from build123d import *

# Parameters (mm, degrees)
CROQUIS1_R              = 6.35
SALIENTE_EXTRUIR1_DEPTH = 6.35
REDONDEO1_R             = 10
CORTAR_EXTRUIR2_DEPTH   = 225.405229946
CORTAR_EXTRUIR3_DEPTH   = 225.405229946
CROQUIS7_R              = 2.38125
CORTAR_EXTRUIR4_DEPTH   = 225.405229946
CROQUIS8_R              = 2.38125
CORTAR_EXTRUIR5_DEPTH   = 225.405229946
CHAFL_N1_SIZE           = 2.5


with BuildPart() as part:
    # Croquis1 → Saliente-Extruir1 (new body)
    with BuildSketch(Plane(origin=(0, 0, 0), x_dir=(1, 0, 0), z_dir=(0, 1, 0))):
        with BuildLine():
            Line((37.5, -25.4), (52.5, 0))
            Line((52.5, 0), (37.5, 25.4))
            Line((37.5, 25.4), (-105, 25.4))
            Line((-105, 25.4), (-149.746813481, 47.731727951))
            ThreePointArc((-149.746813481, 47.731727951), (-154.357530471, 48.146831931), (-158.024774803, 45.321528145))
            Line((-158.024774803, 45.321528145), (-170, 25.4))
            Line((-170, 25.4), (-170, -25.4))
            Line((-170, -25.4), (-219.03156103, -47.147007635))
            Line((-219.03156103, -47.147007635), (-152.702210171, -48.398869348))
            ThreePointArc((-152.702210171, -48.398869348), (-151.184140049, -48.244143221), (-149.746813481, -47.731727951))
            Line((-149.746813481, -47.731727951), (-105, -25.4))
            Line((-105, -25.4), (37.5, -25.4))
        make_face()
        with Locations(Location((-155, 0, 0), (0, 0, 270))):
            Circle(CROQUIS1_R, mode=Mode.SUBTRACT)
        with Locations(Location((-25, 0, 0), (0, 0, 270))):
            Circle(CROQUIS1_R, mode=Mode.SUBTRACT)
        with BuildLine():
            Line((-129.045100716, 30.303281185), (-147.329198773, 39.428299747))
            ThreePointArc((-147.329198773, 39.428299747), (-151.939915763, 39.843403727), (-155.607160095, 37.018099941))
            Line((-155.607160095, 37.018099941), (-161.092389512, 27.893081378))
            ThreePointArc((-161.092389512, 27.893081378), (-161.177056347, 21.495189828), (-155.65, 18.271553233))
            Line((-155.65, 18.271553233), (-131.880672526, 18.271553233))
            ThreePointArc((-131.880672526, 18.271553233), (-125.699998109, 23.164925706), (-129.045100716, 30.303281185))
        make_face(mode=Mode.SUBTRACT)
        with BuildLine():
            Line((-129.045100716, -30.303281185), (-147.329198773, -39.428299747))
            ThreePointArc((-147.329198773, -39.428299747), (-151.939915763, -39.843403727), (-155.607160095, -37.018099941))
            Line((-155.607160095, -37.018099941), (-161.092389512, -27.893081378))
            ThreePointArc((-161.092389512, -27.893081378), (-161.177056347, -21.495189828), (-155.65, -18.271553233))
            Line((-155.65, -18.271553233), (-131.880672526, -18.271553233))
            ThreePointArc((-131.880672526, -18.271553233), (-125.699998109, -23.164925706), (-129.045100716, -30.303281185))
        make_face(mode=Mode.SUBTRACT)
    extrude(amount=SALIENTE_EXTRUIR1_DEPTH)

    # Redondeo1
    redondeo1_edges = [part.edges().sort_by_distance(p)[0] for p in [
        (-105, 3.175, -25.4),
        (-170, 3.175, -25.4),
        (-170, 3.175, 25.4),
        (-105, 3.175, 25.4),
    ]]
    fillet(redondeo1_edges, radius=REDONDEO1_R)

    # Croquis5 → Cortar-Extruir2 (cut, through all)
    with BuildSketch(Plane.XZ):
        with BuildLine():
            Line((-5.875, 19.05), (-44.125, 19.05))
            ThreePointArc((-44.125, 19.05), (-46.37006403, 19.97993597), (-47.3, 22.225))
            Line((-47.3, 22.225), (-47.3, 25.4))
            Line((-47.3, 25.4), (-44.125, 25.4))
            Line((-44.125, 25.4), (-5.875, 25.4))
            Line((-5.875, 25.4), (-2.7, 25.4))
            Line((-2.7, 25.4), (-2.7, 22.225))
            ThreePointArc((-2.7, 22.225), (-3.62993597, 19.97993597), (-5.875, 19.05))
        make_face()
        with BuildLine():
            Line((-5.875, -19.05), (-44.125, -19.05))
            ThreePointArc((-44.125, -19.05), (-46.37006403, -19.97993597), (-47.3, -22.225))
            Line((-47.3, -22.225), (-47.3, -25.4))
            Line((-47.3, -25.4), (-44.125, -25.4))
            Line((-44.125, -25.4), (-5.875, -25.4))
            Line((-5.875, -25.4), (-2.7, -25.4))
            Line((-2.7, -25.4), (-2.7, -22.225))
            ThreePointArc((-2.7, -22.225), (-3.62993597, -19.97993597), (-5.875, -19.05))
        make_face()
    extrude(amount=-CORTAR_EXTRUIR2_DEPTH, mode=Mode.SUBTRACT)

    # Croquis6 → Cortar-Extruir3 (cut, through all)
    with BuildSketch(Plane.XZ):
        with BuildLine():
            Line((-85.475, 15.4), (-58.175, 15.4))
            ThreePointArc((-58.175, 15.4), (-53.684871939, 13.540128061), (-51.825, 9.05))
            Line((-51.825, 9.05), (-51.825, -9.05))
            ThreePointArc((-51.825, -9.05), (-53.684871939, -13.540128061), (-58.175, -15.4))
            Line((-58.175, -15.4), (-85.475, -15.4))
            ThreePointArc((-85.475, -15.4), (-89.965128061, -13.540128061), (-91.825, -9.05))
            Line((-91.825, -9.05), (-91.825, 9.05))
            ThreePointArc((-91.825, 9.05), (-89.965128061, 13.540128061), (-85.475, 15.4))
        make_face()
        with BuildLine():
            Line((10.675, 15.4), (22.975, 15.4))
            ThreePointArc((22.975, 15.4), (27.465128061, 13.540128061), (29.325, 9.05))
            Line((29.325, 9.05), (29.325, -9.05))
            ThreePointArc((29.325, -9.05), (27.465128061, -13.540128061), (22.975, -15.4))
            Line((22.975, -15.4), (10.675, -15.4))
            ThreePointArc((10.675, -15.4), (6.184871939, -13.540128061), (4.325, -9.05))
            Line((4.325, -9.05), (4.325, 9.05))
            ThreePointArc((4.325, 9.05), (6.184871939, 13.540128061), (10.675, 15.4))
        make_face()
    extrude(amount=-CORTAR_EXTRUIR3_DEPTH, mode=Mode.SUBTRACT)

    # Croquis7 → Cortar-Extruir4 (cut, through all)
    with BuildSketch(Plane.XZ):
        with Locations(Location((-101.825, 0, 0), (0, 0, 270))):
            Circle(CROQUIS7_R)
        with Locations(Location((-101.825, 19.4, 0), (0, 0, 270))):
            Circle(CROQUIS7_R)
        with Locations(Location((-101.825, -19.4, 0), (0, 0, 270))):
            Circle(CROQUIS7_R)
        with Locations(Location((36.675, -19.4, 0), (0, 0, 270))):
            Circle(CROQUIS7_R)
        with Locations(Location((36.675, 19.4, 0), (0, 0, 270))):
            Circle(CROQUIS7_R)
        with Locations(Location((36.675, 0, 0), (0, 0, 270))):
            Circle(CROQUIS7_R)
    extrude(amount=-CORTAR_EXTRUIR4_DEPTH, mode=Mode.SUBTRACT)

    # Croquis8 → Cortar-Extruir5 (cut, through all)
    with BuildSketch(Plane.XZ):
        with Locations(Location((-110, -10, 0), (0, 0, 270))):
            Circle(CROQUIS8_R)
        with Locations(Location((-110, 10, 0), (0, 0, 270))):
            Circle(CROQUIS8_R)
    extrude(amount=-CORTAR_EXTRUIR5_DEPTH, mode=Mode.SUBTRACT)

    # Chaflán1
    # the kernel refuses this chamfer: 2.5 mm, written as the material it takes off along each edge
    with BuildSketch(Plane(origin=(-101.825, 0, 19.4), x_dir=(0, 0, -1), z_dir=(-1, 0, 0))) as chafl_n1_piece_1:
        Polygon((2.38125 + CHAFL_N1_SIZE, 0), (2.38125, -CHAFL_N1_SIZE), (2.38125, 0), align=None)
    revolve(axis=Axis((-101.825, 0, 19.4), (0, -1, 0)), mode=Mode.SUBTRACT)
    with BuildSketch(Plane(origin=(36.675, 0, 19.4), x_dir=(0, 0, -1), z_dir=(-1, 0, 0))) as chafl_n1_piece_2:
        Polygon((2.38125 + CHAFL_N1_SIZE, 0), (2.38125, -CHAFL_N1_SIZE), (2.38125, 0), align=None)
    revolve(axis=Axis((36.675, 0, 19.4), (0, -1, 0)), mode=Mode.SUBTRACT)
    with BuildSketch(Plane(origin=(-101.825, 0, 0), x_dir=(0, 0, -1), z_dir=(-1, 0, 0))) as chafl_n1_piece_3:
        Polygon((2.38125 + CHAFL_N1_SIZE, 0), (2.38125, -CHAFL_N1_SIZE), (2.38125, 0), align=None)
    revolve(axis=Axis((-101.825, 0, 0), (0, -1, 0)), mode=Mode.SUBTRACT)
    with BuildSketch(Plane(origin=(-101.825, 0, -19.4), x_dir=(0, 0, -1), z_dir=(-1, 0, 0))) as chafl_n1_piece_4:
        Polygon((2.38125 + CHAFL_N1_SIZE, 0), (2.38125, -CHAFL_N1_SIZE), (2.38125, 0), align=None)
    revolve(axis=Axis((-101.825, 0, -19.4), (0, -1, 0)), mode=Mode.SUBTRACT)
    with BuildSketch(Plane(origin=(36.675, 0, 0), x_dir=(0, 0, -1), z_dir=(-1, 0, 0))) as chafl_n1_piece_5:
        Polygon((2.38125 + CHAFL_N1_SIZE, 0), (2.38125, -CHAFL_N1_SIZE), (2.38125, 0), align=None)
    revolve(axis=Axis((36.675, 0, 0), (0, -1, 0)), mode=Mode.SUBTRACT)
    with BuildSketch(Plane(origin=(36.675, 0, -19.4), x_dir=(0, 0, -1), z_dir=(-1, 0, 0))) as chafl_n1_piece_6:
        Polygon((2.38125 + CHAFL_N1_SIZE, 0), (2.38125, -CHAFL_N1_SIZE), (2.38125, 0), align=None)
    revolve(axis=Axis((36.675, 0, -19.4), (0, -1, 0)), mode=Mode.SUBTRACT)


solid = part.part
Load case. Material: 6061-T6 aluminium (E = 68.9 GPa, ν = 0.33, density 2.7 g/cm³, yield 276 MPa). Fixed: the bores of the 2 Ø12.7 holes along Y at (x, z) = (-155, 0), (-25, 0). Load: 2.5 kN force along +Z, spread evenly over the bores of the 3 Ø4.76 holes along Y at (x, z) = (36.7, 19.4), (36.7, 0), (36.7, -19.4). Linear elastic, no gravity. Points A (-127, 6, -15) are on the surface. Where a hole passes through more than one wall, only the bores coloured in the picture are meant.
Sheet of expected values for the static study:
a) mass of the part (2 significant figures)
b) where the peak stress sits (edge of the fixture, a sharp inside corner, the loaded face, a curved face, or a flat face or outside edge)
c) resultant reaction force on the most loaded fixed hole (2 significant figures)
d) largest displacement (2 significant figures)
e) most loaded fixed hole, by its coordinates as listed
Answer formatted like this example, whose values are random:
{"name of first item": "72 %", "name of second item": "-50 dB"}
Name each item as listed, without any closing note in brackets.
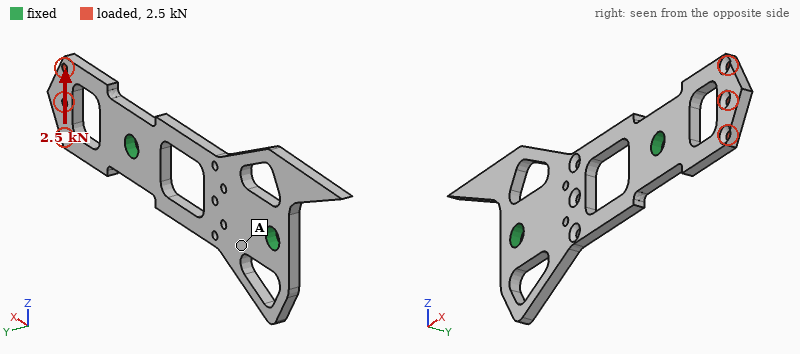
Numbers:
{"mass of the part": "160 g", "where the peak stress sits": "a curved face", "resultant reaction force on the most loaded fixed hole": "2.7 kN", "largest displacement": "0.40 mm", "most loaded fixed hole, by its coordinates as listed": "(-25, 0)"}
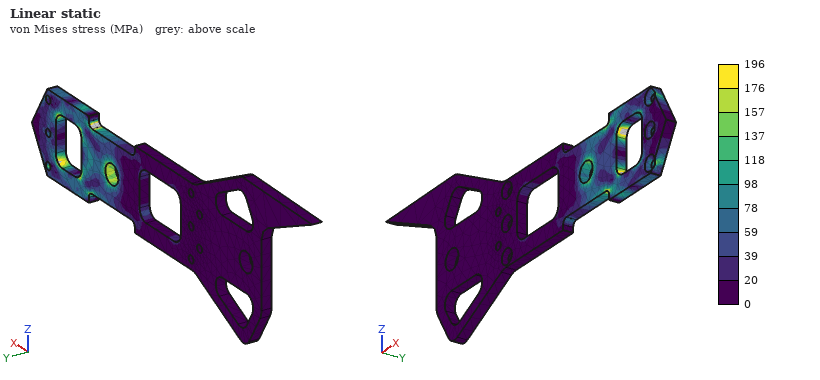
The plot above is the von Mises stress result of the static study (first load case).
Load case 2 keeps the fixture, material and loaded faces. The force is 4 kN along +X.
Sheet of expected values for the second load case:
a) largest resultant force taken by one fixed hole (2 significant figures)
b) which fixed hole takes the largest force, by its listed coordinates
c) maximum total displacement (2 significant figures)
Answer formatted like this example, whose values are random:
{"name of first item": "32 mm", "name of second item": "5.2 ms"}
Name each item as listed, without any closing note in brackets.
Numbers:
{"largest resultant force taken by one fixed hole": "3.9 kN", "which fixed hole takes the largest force, by its listed coordinates": "(-25, 0)", "maximum total displacement": "0.34 mm"}
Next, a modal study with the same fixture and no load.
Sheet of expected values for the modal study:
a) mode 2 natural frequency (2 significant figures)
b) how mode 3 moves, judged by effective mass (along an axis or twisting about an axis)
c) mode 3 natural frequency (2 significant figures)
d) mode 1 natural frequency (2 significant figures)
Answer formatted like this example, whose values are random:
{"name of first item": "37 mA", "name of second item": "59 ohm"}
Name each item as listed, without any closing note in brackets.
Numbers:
{"mode 2 natural frequency": "1300 Hz", "how mode 3 moves, judged by effective mass": "along Y", "mode 3 natural frequency": "2000 Hz", "mode 1 natural frequency": "1000 Hz"}
